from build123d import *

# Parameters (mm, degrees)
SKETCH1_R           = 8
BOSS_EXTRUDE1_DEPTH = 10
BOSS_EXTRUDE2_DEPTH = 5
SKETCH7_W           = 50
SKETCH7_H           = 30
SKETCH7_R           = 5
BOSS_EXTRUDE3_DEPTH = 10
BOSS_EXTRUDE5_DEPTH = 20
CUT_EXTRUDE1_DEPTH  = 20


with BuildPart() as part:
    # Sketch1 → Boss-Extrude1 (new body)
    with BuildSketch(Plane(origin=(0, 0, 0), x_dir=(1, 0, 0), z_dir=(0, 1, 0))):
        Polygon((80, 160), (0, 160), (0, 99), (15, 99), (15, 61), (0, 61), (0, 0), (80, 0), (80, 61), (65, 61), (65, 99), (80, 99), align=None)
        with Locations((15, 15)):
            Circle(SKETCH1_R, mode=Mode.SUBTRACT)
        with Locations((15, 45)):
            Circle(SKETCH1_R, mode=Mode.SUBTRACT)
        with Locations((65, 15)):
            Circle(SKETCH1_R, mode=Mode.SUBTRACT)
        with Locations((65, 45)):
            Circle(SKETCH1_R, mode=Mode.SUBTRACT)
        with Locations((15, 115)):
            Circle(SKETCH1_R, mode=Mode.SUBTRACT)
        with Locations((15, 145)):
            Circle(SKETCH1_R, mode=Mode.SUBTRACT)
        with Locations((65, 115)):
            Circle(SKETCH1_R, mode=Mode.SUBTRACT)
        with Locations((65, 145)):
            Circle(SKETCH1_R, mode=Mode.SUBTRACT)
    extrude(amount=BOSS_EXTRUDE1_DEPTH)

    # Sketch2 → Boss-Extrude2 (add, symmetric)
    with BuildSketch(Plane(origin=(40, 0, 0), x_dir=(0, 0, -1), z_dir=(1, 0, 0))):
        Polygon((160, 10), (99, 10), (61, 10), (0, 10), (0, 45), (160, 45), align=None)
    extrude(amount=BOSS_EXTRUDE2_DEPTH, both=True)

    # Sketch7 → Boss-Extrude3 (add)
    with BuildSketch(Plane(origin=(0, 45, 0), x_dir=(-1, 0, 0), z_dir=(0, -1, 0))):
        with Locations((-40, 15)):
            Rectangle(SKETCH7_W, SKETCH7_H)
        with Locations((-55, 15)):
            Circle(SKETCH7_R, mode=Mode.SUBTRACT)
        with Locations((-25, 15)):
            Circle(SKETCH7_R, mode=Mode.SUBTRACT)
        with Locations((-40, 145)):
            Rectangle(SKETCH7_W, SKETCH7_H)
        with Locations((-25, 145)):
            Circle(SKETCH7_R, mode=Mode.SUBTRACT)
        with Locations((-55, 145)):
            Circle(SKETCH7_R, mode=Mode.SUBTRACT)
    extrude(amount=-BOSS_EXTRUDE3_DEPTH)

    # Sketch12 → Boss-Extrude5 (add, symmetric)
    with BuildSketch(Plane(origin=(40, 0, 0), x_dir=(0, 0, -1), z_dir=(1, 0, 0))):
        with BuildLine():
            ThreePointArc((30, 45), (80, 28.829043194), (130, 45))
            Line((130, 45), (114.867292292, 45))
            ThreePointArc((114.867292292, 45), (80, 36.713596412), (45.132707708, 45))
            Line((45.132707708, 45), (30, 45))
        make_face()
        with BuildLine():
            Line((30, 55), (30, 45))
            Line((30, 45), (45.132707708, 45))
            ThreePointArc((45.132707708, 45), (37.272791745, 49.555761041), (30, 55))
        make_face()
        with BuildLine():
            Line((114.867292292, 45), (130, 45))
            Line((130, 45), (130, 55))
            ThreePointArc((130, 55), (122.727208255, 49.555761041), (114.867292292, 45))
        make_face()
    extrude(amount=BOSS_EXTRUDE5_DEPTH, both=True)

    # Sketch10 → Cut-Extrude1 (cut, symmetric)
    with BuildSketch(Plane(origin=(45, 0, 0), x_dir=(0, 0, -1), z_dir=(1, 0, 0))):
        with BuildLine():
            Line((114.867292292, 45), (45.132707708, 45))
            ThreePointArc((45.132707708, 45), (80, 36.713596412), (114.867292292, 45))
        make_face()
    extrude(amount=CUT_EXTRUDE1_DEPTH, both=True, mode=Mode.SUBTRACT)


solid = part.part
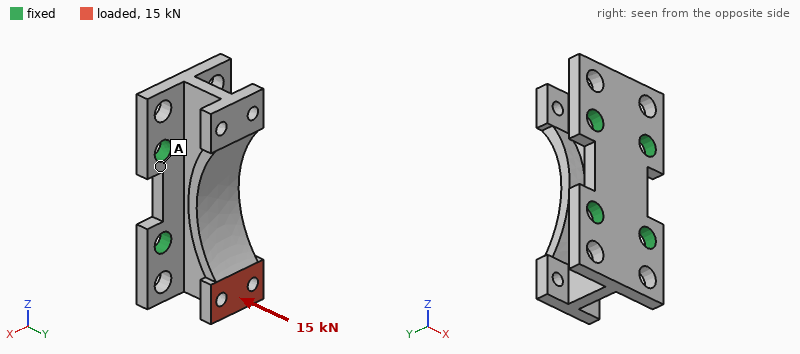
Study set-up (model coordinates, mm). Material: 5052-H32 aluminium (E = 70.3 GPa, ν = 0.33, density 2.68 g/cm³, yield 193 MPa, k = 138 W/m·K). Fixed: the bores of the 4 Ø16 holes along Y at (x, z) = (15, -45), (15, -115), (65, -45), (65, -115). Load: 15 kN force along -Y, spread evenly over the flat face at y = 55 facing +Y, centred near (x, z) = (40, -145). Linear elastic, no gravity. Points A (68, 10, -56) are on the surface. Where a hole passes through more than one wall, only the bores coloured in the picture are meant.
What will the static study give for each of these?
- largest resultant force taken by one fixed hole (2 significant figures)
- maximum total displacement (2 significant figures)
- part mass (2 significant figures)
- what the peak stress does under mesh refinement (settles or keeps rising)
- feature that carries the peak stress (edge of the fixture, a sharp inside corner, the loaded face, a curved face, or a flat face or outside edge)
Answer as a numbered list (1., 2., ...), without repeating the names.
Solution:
1. 10 kN
2. 0.25 mm
3. 550 g
4. keeps rising
5. edge of the fixture
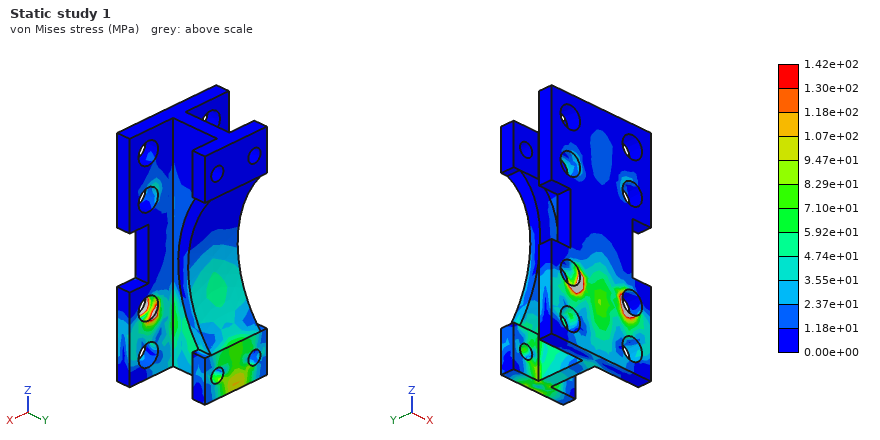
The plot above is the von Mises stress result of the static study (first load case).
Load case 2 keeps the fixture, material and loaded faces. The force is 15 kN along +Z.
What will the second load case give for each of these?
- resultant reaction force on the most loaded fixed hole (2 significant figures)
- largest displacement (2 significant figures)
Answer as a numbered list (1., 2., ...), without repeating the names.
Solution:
1. 6.9 kN
2. 0.21 mm
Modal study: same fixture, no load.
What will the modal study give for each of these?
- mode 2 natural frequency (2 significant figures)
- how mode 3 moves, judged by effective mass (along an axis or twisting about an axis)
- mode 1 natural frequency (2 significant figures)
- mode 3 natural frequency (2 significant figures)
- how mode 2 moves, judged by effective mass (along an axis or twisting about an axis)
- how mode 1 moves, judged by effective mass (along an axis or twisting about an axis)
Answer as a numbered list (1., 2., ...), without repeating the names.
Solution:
1. 2400 Hz
2. along Z
3. 2200 Hz
4. 4200 Hz
5. twisting about Y
6. along X
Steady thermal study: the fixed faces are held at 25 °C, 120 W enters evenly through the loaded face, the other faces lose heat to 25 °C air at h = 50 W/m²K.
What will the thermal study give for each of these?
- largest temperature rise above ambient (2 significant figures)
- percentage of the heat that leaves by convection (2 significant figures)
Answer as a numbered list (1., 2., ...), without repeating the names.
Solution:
1. 73 K
2. 25 %
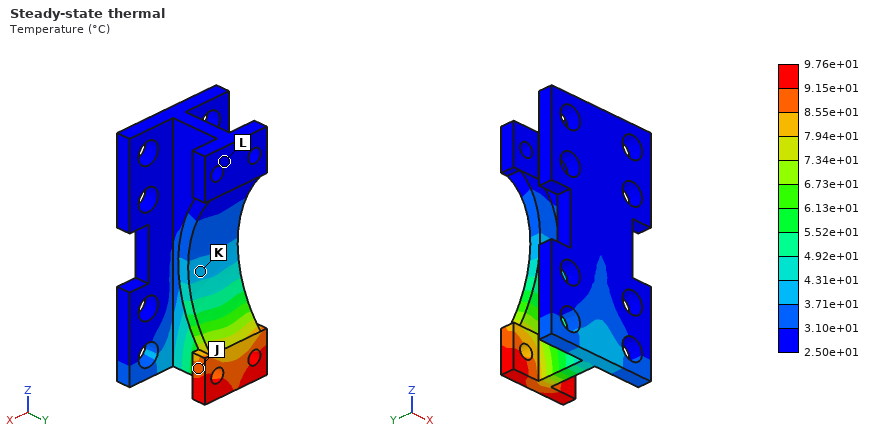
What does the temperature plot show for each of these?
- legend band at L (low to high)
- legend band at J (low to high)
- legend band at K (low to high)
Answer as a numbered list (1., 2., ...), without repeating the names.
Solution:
1. 2.50e+01 to 3.10e+01 °C
2. 8.55e+01 to 9.15e+01 °C
3. 3.71e+01 to 4.31e+01 °C
